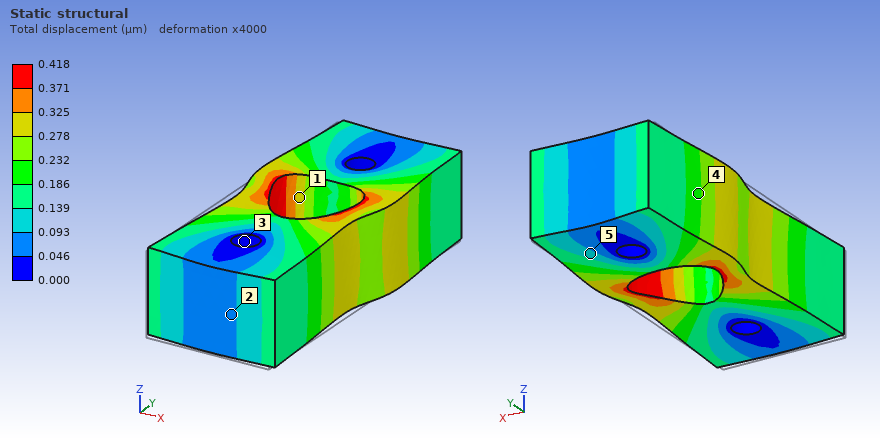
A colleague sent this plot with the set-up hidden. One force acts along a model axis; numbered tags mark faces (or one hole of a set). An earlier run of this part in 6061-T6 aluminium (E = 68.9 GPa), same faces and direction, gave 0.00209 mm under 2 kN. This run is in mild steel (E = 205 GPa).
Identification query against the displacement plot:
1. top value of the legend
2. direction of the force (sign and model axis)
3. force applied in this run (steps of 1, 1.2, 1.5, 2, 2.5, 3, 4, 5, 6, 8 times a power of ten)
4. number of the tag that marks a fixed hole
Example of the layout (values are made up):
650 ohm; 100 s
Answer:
0.418 µm; +Y; 1.2 kN; 3
